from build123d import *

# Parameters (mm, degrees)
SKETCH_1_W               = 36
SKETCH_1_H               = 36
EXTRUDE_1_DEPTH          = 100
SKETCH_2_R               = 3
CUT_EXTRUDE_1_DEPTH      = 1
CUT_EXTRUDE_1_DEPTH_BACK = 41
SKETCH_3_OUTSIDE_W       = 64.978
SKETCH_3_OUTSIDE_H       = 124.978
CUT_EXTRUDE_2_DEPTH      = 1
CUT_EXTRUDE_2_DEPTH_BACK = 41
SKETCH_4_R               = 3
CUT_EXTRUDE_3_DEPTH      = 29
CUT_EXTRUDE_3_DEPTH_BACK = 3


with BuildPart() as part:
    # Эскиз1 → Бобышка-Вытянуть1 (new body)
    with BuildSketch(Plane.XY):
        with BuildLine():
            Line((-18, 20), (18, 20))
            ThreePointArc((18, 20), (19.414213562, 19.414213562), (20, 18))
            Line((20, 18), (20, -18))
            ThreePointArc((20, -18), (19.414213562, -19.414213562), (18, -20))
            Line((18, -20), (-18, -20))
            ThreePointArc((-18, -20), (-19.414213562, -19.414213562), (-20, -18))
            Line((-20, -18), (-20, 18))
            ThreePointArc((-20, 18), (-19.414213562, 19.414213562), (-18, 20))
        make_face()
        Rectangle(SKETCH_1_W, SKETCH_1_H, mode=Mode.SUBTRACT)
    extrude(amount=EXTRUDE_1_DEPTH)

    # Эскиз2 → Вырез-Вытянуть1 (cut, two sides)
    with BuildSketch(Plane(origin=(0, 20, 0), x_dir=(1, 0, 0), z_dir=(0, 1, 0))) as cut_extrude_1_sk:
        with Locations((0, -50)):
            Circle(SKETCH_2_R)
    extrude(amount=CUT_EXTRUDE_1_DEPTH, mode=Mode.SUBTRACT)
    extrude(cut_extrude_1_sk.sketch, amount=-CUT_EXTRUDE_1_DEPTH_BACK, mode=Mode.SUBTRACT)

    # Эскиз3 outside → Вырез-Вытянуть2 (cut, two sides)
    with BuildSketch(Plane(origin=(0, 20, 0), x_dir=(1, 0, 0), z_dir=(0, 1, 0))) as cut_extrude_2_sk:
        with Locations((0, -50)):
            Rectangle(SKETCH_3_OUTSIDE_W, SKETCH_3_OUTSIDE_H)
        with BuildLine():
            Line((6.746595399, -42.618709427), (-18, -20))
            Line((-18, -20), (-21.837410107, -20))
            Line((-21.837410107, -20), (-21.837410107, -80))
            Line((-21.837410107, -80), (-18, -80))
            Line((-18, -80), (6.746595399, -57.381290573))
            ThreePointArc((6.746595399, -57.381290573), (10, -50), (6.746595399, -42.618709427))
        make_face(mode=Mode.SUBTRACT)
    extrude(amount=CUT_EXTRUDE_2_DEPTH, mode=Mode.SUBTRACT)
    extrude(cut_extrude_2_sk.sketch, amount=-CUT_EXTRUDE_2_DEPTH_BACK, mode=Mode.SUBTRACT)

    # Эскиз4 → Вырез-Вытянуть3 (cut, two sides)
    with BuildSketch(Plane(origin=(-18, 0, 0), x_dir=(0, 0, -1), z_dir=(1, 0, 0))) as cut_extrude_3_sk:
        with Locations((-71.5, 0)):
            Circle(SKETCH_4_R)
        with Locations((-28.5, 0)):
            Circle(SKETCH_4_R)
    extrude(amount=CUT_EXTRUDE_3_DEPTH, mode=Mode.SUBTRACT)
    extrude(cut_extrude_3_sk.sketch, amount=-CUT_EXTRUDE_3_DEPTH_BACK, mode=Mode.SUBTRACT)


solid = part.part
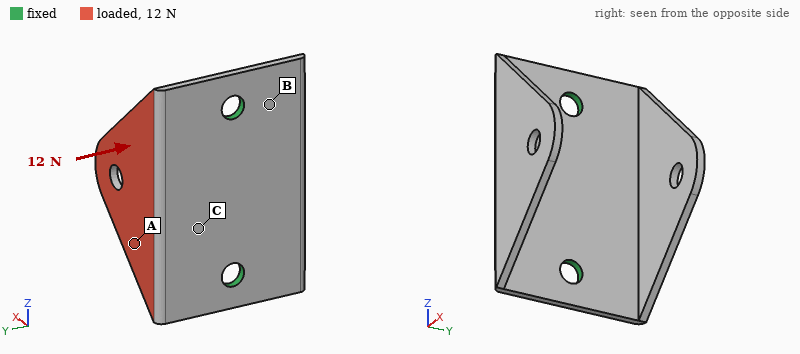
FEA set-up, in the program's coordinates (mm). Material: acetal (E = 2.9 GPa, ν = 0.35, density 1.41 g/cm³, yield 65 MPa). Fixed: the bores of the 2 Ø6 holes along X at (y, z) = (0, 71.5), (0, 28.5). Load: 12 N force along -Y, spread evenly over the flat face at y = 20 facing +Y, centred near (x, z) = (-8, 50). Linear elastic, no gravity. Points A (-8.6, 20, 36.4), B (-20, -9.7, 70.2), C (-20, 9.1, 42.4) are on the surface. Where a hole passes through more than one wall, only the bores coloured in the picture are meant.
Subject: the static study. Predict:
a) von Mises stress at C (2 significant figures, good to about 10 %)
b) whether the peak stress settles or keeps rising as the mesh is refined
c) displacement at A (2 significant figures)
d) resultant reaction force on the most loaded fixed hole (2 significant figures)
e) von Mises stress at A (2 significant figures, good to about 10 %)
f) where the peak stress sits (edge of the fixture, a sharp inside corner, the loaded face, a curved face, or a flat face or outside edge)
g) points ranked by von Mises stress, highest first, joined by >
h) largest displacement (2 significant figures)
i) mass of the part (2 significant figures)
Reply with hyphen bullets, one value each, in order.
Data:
- 2.6 MPa
- keeps rising
- 0.32 mm
- 6.1 N
- 1.7 MPa
- edge of the fixture
- C > A > B
- 0.86 mm
- 12 g
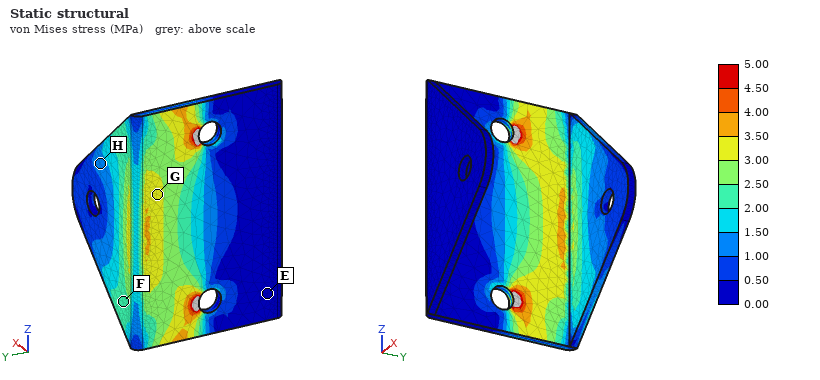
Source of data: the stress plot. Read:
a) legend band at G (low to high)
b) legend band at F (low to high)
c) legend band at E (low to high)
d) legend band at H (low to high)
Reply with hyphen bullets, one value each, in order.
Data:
- 3.00 to 3.50 MPa
- 2.00 to 2.50 MPa
- 0.00 to 0.50 MPa
- 1.00 to 1.50 MPa
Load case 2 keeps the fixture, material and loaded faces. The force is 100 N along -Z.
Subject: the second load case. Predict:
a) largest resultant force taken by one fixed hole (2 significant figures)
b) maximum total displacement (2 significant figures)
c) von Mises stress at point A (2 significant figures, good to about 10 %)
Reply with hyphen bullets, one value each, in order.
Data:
- 70 N
- 0.79 mm
- 3.4 MPa
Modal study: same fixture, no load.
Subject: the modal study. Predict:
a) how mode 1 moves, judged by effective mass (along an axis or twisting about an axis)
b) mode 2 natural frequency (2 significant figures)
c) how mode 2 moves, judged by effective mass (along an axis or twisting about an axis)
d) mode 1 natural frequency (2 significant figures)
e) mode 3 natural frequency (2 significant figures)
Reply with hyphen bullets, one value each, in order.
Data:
- along Y
- 450 Hz
- along X
- 420 Hz
- 910 Hz
